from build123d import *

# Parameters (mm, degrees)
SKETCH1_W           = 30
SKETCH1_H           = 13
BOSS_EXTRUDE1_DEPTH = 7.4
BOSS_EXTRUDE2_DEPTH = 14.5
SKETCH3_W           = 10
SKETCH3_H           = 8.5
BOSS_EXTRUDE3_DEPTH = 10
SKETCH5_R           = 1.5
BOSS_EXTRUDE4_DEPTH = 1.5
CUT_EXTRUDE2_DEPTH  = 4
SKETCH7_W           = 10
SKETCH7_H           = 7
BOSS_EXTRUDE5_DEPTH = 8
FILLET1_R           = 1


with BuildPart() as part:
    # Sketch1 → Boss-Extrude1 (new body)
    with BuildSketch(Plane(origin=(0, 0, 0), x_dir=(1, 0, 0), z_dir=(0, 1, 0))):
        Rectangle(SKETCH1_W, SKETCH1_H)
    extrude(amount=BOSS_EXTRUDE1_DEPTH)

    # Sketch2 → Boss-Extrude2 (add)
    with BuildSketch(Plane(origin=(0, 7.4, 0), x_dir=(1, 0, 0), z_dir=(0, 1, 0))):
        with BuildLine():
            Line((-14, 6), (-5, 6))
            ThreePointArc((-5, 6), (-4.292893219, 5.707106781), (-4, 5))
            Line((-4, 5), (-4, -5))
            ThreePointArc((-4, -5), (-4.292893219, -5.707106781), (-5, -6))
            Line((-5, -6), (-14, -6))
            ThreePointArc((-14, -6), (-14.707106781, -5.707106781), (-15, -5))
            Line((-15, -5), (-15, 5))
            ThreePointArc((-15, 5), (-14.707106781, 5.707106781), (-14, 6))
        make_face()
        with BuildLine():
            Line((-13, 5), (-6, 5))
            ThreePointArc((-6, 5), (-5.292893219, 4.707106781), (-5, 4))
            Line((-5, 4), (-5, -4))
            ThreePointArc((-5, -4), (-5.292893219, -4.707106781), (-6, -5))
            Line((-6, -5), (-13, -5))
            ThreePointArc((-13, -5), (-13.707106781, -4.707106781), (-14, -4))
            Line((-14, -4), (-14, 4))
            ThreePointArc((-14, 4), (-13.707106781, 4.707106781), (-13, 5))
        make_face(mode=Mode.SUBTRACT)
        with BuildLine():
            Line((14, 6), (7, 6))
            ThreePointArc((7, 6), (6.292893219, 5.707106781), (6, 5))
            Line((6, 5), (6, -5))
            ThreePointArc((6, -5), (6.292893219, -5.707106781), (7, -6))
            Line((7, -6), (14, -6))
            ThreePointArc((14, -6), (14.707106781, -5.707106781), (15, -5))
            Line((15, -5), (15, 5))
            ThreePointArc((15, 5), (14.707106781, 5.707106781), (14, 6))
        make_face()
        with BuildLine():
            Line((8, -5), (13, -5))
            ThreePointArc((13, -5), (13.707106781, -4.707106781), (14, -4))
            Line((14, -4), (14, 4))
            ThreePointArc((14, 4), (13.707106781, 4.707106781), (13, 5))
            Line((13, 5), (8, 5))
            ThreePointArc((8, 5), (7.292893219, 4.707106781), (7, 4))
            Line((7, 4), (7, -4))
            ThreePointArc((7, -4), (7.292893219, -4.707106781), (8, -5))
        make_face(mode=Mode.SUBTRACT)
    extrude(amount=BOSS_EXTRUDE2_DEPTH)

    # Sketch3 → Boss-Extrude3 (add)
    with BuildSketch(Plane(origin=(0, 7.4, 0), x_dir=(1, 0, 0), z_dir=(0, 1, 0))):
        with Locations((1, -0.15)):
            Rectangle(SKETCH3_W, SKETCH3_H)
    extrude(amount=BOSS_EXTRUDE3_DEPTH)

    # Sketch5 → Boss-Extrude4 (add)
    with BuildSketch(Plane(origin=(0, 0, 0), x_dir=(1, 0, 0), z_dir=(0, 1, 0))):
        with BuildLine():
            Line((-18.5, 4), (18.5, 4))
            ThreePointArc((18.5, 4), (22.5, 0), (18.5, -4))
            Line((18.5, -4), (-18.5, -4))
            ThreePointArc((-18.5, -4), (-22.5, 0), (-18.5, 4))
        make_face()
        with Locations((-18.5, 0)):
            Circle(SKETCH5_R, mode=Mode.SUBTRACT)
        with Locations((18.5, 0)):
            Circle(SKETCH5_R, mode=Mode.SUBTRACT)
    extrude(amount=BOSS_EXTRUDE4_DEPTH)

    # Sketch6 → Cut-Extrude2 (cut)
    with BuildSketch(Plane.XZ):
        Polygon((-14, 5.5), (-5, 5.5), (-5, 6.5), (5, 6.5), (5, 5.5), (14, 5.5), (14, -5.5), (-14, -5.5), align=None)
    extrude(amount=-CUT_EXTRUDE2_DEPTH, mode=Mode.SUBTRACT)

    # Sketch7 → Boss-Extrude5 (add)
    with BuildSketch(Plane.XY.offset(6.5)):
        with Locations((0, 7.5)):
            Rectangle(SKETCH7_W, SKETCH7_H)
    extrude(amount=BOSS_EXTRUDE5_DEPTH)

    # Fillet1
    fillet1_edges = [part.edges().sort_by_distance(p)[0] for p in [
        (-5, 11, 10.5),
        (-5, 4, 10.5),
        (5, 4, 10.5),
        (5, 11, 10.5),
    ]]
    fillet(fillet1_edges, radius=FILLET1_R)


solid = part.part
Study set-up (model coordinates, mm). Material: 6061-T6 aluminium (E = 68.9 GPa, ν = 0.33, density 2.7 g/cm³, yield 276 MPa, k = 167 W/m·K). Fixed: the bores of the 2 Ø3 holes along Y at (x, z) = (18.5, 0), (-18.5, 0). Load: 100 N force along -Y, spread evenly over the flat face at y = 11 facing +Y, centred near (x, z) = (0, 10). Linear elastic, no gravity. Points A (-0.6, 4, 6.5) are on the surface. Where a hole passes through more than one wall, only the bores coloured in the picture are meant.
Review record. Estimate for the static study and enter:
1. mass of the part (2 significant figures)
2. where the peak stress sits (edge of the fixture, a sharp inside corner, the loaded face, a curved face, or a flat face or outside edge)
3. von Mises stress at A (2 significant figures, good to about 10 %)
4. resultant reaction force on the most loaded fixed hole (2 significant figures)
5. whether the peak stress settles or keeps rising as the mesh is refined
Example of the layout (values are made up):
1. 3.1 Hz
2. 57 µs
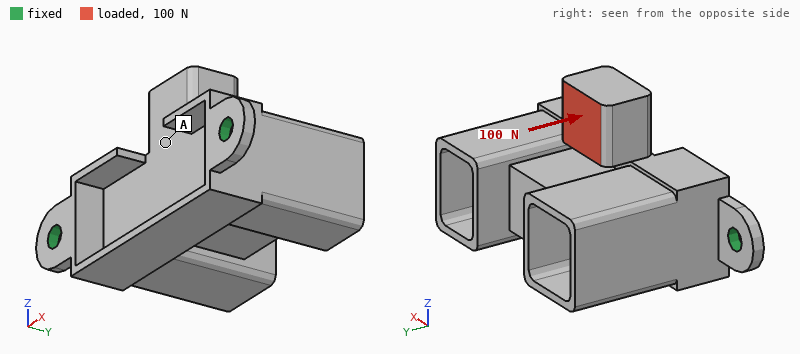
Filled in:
1. 12 g
2. edge of the fixture
3. 15 MPa
4. 59 N
5. keeps rising
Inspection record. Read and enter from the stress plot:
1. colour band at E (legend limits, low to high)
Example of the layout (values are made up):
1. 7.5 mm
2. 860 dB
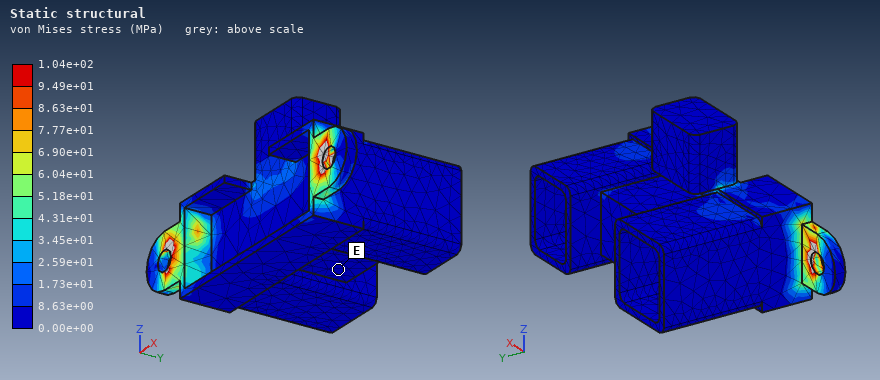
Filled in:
1. 0.00e+00 to 8.63e+00 MPa
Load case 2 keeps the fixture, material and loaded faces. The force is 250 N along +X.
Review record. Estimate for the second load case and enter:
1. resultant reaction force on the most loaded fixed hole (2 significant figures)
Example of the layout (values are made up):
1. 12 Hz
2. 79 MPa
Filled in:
1. 170 N
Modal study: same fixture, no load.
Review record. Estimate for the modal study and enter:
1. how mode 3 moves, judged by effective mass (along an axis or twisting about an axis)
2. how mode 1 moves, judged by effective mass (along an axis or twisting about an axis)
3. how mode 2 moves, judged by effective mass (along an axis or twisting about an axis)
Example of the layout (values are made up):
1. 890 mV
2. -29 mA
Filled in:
1. along X
2. along Z
3. along Y
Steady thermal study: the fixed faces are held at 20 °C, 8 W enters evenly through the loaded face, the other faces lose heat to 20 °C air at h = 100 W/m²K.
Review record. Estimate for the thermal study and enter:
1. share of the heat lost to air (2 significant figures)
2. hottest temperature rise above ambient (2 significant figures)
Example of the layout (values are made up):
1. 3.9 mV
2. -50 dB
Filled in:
1. 45 %
2. 19 K
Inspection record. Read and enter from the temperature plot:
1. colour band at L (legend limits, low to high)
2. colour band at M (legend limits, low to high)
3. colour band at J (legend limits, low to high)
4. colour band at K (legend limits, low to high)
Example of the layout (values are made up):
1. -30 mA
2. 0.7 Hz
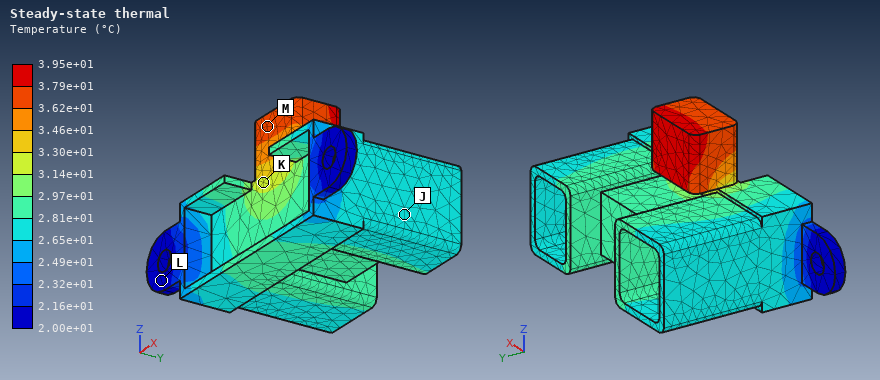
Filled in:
1. 2.00e+01 to 2.16e+01 °C
2. 3.62e+01 to 3.79e+01 °C
3. 2.65e+01 to 2.81e+01 °C
4. 3.14e+01 to 3.30e+01 °C
